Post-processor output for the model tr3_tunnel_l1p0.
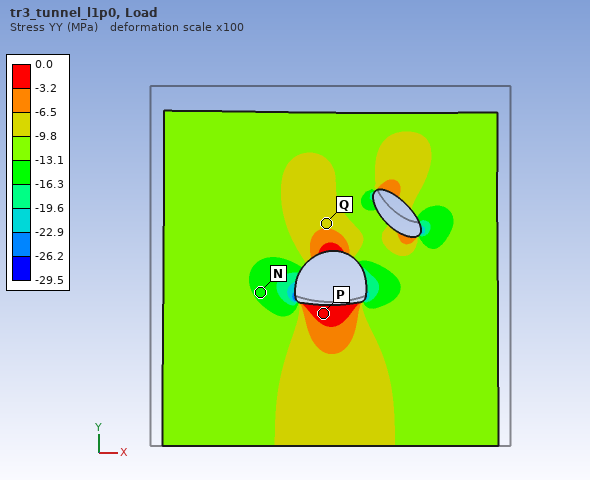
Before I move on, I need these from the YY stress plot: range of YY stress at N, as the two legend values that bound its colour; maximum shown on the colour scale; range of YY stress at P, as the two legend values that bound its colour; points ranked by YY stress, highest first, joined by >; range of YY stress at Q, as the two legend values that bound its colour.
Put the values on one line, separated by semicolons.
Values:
-16.3 to -13.1 MPa; 0.0 MPa; -3.2 to 0.0 MPa; P > Q > N; -9.8 to -6.5 MPa
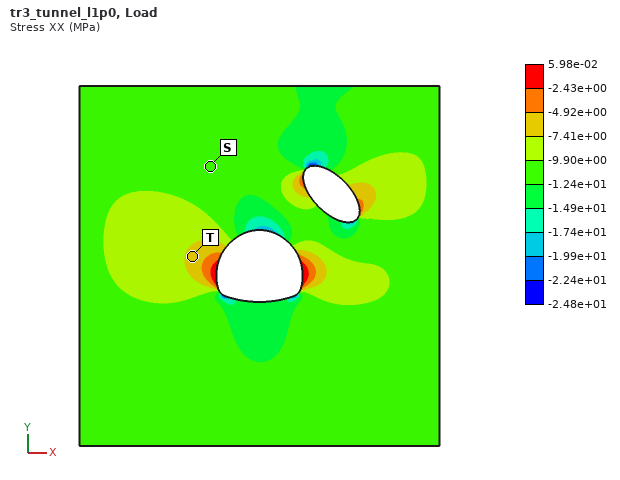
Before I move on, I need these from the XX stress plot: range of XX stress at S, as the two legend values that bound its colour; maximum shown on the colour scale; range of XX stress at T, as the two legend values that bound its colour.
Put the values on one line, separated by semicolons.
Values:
-1.24e+01 to -9.90e+00 MPa; 5.98e-02 MPa; -7.41e+00 to -4.92e+00 MPa
